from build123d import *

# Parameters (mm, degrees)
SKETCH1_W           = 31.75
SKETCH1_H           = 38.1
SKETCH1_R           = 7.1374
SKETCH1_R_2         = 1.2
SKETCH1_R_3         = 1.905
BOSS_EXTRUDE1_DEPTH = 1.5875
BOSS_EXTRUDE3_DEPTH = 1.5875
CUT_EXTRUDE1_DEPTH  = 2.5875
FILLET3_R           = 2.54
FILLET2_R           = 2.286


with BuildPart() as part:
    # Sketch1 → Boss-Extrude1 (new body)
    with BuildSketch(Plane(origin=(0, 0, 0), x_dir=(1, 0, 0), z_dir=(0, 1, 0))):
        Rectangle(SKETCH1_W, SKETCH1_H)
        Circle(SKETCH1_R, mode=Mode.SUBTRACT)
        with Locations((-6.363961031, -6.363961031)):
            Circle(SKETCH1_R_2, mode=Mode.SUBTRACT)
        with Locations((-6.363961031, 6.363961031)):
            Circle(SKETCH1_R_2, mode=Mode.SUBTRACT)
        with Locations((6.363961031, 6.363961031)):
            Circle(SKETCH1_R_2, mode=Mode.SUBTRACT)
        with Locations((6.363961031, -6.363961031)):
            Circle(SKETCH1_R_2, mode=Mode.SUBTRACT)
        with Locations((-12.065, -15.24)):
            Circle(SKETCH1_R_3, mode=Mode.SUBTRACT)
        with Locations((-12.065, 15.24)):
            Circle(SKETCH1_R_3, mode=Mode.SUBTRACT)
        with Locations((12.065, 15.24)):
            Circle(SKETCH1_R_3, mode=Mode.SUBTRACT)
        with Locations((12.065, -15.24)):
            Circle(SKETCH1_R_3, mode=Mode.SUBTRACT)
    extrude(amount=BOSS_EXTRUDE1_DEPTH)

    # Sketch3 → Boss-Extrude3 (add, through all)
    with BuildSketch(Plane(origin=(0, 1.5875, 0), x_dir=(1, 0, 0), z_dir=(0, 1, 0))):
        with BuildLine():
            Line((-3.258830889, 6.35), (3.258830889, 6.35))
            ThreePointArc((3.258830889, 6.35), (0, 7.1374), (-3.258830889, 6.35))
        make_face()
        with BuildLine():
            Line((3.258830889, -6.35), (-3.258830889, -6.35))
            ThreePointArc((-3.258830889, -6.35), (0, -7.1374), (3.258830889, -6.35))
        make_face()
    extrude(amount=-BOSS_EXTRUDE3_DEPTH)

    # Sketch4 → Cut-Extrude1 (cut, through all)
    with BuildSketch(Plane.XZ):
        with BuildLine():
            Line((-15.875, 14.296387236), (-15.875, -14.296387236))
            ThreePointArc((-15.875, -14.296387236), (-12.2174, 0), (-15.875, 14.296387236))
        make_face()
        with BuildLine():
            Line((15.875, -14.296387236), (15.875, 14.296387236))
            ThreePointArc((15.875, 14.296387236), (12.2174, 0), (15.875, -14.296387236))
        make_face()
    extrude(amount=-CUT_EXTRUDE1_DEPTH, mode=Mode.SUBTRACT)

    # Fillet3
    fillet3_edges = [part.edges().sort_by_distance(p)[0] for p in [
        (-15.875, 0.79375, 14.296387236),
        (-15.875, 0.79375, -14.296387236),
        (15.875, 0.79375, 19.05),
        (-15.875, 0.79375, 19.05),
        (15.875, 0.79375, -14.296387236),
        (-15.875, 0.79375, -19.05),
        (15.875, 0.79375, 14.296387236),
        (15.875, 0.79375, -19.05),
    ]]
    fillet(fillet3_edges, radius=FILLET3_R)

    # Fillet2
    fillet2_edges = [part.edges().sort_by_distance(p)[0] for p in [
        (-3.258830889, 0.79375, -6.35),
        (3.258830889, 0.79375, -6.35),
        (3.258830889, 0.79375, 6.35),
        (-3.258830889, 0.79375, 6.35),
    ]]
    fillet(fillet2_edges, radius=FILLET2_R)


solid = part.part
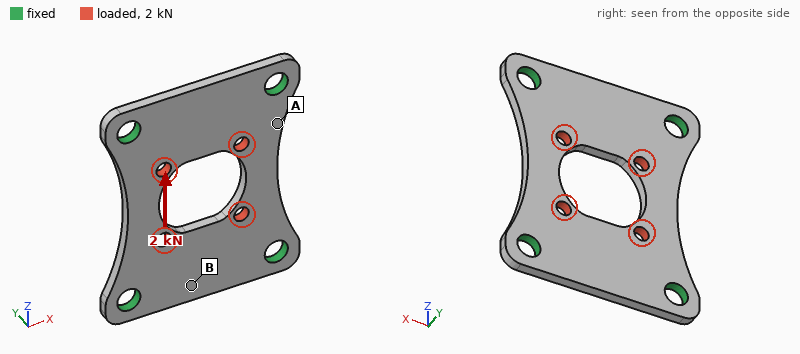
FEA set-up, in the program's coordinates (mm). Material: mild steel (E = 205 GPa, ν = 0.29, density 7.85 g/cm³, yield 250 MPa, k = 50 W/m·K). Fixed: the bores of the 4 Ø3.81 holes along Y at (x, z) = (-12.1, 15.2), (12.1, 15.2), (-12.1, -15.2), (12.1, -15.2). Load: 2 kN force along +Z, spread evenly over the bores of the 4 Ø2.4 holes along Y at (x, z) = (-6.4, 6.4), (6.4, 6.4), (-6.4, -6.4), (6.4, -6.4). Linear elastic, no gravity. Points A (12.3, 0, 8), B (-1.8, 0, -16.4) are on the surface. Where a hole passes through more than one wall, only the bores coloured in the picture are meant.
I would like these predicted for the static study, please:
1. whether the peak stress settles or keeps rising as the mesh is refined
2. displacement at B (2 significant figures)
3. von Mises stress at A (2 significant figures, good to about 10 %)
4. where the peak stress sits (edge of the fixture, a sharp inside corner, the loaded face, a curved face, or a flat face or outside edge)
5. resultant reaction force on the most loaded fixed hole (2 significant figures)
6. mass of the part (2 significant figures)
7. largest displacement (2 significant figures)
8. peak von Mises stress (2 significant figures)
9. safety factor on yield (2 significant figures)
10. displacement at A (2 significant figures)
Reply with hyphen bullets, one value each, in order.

- settles
- 2.0 µm
- 29 MPa
- the loaded face
- 530 N
- 11 g
- 3.2 µm
- 120 MPa
- 2.1
- 0.88 µm
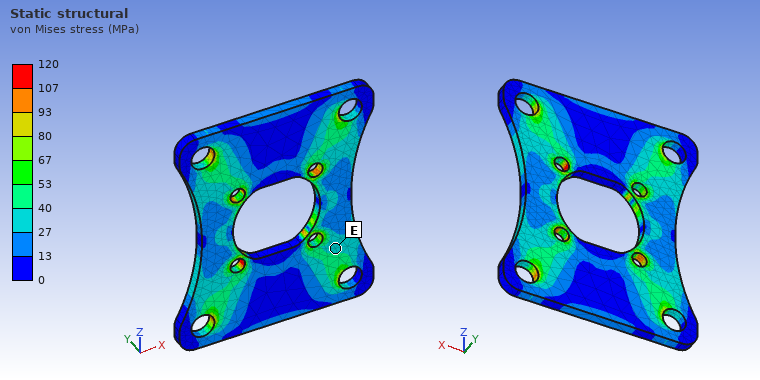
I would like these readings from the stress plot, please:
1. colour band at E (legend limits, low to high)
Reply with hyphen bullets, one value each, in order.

- 27 to 40 MPa
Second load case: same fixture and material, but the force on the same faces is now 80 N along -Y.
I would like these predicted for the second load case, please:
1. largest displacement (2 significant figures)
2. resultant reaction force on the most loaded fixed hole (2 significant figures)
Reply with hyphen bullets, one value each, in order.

- 7.1 µm
- 20 N
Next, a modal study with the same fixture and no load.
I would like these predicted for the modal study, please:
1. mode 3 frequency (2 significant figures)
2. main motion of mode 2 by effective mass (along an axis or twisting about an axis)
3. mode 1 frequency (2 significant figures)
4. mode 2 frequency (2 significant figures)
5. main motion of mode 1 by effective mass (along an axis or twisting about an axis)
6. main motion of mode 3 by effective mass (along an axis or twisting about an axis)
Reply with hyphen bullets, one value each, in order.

- 16 kHz
- twisting about Z
- 10 kHz
- 14 kHz
- along Y
- twisting about X
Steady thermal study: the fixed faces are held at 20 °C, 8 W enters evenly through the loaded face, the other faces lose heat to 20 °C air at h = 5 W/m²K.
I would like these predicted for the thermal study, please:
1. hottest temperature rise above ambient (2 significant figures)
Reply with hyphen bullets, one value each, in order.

- 27 K
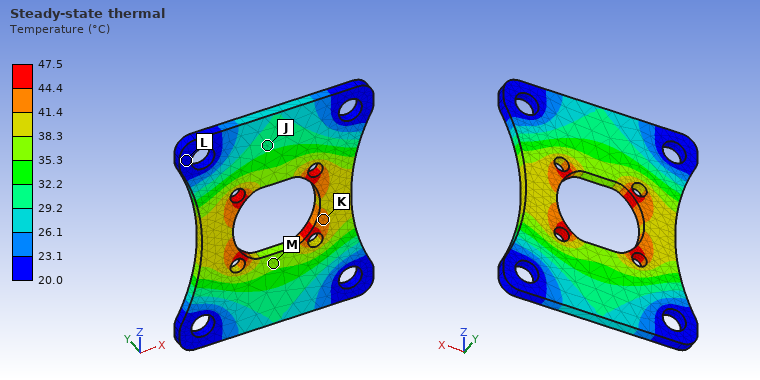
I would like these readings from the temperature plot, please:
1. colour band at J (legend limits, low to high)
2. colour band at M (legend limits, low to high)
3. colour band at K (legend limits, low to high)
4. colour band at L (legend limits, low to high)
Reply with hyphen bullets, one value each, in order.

- 29.2 to 32.2 °C
- 35.3 to 38.3 °C
- 41.4 to 44.4 °C
- 20.0 to 23.1 °C
